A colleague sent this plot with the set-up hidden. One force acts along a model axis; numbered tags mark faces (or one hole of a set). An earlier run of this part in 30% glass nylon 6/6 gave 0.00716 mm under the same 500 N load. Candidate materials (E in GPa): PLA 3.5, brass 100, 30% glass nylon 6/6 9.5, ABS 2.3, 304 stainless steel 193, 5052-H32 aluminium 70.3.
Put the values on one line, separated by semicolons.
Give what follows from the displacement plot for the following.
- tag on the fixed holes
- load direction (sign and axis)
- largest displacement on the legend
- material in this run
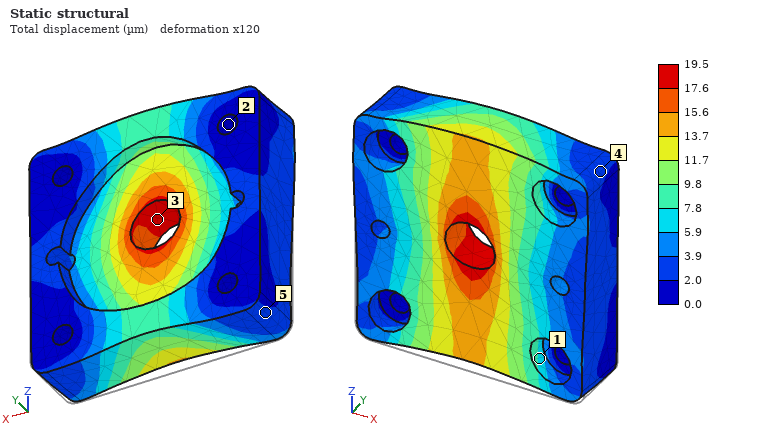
2; +Z; 19.5 µm; PLA
